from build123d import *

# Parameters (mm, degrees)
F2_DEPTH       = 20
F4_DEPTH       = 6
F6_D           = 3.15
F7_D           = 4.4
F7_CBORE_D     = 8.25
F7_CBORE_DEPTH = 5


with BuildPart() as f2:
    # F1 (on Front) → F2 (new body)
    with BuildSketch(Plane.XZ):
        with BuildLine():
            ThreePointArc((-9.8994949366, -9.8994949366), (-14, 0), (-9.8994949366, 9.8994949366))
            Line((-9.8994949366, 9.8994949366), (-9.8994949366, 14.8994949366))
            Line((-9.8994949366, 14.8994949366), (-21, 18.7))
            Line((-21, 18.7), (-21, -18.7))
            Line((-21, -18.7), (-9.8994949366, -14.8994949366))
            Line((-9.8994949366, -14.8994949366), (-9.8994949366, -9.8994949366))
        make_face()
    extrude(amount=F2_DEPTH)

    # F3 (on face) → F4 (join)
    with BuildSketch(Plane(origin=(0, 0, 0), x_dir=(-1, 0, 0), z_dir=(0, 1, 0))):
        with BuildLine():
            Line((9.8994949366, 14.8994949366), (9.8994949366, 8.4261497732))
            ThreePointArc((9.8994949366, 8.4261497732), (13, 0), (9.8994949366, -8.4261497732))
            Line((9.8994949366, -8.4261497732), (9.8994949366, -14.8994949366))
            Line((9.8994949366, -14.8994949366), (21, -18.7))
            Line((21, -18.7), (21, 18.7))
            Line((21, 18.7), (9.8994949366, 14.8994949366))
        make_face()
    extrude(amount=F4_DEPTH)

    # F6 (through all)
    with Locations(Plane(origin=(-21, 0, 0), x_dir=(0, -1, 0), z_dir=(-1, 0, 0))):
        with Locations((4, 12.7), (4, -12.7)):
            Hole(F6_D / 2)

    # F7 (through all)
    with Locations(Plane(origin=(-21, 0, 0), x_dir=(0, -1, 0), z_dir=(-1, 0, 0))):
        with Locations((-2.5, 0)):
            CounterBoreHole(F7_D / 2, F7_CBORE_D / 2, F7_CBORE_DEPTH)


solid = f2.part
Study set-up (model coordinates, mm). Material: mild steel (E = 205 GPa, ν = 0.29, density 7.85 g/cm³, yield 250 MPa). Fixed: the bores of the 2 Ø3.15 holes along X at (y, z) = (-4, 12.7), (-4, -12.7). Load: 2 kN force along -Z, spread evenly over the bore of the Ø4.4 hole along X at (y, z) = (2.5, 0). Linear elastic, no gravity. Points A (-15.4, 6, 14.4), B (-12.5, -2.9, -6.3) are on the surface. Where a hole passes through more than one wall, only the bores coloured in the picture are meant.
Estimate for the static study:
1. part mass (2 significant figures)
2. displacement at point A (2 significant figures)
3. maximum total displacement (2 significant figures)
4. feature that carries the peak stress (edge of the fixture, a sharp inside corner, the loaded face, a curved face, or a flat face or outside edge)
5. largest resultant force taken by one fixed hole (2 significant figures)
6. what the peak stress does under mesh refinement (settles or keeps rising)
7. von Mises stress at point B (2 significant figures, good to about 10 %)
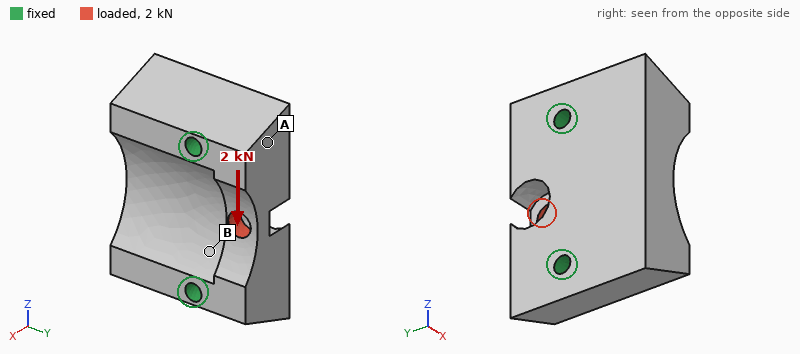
62 g
0.96 µm
2.5 µm
a sharp inside corner
1.1 kN
keeps rising
16 MPa
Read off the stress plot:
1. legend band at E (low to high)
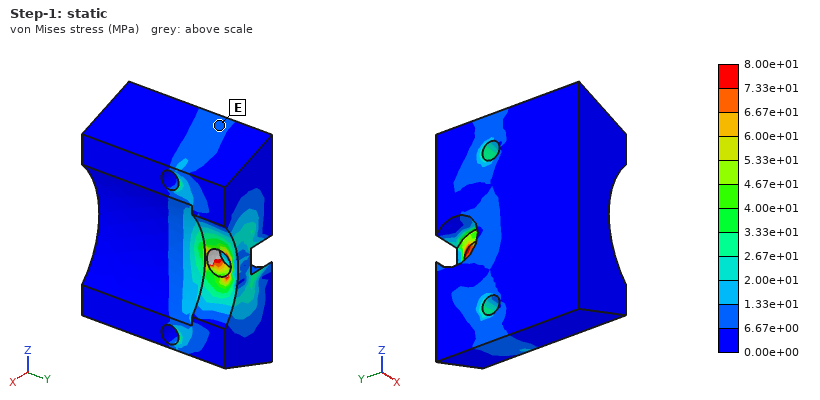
6.67e+00 to 1.33e+01 MPa
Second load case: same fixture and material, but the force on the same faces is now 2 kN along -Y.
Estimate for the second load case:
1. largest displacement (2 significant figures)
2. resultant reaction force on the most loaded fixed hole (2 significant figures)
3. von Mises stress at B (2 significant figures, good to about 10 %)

6.6 µm
1.0 kN
28 MPa
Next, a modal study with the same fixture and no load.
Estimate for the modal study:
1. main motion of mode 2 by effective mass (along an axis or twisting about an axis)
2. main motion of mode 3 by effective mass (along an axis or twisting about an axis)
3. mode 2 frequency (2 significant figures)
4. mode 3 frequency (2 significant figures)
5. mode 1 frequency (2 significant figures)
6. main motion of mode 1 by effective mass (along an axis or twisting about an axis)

twisting about Y
along Z
31 kHz
39 kHz
23 kHz
along X
